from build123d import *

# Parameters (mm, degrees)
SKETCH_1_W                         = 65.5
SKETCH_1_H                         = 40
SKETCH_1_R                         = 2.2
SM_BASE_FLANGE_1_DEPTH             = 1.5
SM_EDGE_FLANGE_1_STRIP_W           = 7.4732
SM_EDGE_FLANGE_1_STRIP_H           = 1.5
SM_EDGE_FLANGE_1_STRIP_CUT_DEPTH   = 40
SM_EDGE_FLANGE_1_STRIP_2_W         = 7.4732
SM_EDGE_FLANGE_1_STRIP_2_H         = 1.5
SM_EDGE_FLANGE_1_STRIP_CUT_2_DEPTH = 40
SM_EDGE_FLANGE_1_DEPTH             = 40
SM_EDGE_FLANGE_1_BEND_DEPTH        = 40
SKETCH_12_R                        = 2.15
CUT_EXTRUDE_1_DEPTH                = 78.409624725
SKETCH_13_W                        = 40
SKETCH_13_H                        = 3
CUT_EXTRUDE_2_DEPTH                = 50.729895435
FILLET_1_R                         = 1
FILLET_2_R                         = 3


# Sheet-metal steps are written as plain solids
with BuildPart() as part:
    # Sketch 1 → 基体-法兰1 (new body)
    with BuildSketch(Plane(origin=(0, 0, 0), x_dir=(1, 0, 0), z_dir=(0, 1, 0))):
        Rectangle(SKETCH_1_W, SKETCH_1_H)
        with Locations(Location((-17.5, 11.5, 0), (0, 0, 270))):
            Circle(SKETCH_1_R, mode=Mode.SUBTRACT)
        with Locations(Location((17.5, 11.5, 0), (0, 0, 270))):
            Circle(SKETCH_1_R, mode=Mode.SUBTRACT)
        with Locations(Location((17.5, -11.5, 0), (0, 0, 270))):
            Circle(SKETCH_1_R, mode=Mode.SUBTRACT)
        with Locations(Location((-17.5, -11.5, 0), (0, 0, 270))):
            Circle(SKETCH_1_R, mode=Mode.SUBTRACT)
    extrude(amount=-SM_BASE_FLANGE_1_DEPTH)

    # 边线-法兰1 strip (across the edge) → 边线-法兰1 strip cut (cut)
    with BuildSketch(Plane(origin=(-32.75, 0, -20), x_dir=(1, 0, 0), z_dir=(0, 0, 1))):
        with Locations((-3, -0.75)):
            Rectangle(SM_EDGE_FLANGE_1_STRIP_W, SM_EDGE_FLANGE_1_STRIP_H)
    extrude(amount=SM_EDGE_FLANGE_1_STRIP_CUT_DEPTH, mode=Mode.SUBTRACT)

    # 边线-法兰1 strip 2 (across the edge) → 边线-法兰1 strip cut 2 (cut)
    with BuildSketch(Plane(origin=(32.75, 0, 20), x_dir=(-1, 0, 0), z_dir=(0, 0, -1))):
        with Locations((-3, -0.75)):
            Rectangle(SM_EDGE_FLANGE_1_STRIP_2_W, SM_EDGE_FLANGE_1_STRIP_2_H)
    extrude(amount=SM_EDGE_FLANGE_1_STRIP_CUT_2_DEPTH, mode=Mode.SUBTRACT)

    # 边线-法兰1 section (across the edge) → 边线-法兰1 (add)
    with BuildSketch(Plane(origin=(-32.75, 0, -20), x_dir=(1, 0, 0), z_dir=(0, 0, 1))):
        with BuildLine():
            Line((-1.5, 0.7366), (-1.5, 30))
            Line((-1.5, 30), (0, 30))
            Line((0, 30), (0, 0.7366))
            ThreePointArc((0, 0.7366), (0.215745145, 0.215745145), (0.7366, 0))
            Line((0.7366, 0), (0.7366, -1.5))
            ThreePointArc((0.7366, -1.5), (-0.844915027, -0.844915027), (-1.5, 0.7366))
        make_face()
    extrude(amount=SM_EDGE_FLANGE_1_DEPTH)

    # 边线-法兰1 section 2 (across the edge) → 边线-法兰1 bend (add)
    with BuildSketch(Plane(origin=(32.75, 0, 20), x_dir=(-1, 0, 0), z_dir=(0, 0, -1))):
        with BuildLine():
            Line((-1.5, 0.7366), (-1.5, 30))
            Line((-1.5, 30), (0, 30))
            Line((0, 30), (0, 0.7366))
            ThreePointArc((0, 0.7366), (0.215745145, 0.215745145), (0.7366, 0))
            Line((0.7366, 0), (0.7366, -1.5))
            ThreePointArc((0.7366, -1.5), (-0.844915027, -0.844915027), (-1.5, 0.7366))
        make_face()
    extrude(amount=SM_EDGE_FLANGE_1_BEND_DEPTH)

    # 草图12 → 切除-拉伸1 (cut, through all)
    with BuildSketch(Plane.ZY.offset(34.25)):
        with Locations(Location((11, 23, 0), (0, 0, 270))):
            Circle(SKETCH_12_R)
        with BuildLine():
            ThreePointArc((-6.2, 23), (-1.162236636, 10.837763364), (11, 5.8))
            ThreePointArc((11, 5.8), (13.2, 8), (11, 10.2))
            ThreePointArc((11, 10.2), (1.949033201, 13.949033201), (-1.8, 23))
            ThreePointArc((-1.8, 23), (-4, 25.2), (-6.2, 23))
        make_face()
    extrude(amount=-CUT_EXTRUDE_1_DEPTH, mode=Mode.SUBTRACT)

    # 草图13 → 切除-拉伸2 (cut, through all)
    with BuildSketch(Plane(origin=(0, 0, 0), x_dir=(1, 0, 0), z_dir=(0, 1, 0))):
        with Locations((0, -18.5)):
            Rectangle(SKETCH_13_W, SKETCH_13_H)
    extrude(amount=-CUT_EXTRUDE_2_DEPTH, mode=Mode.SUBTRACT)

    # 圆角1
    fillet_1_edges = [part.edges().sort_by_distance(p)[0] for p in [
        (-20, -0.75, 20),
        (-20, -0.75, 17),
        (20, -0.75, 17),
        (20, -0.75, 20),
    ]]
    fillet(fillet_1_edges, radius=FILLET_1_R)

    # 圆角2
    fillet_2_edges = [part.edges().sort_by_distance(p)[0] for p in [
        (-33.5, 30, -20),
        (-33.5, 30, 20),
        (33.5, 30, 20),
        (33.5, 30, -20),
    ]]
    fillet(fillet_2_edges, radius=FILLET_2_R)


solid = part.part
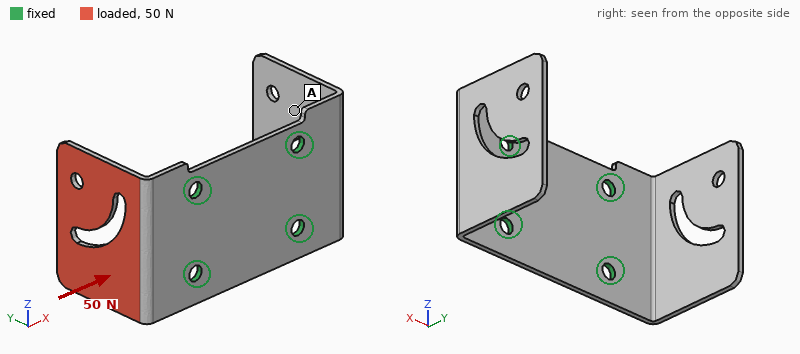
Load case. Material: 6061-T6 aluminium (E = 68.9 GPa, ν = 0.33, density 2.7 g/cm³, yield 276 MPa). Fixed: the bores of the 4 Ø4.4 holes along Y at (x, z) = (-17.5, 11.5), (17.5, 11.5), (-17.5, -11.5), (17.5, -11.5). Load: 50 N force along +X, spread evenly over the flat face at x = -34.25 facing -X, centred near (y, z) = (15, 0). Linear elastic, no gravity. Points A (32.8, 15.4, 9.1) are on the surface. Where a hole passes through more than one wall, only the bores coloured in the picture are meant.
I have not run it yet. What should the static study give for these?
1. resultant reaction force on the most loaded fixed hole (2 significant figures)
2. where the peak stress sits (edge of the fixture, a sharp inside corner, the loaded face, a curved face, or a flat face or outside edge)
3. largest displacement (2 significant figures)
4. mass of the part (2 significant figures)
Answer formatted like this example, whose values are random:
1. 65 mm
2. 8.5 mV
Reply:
1. 23 N
2. a flat face or outside edge
3. 0.79 mm
4. 19 g
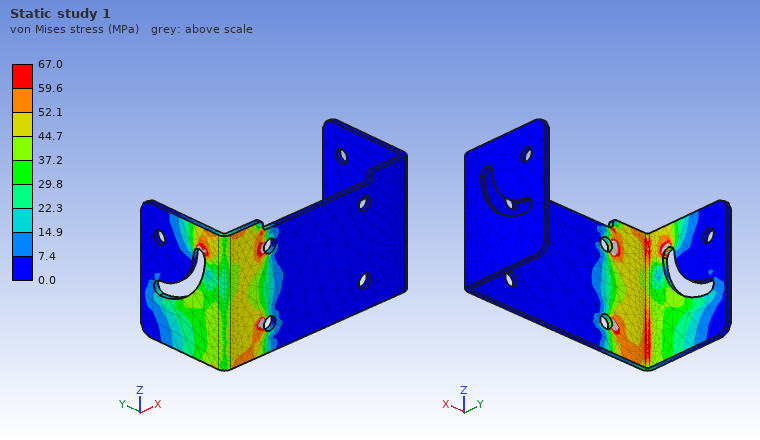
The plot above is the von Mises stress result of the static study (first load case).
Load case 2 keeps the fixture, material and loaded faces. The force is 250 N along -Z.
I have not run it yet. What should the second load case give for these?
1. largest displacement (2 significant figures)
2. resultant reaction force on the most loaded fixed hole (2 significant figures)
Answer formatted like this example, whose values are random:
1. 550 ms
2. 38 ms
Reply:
1. 0.64 mm
2. 250 N
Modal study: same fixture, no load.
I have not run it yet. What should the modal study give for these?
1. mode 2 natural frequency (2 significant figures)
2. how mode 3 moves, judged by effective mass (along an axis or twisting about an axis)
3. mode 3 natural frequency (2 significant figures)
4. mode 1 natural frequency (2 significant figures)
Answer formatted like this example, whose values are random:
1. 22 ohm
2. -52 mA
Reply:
1. 740 Hz
2. along Z
3. 1500 Hz
4. 740 Hz
